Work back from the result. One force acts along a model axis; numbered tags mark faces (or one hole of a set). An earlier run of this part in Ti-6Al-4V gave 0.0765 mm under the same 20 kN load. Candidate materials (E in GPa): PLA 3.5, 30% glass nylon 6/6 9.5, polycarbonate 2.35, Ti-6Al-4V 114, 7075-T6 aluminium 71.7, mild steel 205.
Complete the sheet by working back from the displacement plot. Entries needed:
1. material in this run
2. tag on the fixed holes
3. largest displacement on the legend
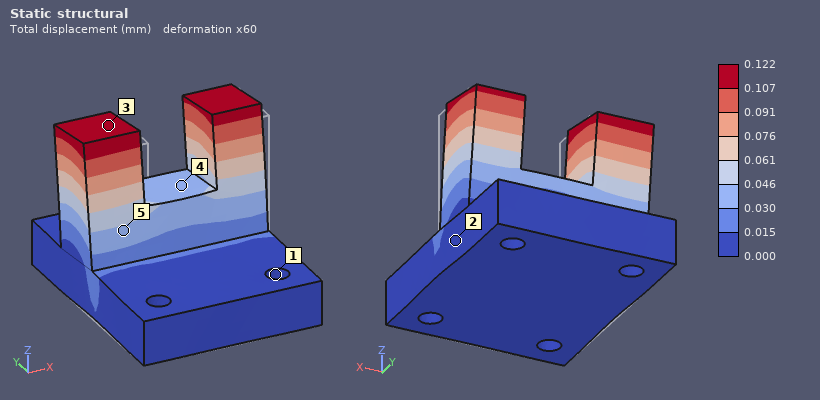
7075-T6 aluminium
1
0.122 mm
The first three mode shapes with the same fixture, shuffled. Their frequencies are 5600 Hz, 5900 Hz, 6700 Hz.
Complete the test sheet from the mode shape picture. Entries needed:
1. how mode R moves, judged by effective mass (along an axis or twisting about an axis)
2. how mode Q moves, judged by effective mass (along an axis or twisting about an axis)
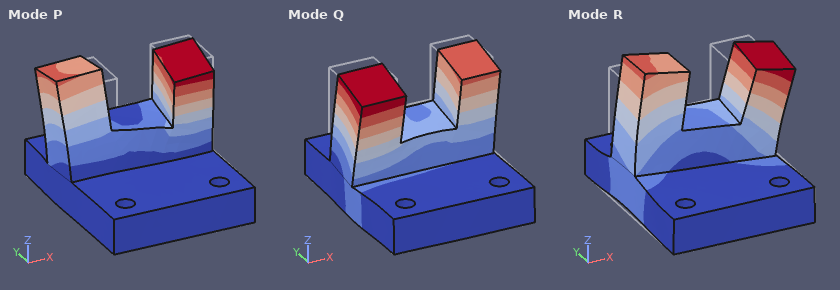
along X
along Y
